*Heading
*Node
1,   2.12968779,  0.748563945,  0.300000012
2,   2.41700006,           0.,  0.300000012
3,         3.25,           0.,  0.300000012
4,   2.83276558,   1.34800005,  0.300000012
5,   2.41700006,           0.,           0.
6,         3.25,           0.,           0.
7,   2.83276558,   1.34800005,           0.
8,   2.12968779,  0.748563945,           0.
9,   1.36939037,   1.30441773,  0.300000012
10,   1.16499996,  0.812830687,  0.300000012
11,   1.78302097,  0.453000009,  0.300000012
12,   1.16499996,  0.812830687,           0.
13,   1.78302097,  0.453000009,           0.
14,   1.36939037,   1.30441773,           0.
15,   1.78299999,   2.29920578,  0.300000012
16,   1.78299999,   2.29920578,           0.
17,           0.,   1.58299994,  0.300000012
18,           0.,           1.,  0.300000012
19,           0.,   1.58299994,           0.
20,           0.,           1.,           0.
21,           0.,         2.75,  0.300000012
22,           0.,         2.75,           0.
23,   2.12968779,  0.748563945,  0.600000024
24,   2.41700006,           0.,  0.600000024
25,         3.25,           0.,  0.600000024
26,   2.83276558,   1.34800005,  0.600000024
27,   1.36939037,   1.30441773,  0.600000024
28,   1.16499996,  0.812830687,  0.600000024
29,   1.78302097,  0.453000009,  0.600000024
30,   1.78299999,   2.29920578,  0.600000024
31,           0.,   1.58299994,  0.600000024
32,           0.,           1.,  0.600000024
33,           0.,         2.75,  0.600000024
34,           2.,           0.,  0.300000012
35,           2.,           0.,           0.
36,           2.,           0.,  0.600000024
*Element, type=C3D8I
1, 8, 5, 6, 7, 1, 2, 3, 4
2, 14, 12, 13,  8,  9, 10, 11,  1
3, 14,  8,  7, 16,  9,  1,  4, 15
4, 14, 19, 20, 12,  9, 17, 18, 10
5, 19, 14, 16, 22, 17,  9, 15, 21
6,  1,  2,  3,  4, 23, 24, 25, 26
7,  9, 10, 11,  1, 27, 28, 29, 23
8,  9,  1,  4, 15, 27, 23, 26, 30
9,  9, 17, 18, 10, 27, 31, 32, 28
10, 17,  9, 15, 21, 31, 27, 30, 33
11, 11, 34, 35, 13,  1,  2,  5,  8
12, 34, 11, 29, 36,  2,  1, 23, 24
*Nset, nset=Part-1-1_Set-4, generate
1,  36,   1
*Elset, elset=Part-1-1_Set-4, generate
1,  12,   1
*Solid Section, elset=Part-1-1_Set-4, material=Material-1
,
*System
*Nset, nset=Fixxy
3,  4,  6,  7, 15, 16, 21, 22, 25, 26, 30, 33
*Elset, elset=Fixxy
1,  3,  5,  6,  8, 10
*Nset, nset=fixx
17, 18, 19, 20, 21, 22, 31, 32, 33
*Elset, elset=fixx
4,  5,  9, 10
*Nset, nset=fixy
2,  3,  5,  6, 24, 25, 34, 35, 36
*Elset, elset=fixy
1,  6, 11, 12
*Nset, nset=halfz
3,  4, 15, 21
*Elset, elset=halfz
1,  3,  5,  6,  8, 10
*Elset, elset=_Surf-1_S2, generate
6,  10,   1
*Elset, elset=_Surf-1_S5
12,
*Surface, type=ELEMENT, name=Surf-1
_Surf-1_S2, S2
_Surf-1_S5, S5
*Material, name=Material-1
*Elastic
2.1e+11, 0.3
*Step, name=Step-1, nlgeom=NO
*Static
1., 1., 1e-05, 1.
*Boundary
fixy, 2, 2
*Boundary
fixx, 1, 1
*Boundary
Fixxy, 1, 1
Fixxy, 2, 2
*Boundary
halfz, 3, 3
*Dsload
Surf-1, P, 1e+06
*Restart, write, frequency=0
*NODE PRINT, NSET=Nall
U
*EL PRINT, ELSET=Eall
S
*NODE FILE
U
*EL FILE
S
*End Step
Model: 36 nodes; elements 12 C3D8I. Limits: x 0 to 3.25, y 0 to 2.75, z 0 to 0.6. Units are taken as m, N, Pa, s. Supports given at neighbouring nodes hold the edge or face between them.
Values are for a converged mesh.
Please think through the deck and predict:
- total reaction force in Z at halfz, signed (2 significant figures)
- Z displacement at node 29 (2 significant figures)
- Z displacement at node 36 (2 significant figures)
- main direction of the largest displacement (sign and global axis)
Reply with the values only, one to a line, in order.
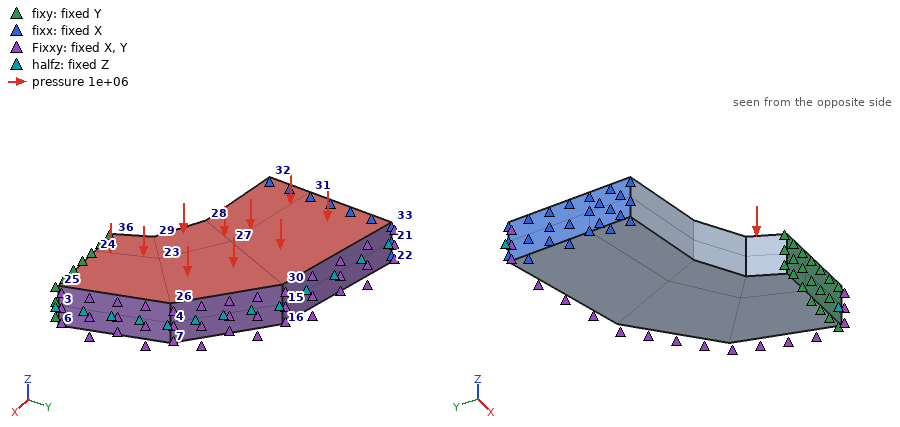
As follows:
5.2e+06 N
-1.0e-04 m
-8.6e-05 m
-Z
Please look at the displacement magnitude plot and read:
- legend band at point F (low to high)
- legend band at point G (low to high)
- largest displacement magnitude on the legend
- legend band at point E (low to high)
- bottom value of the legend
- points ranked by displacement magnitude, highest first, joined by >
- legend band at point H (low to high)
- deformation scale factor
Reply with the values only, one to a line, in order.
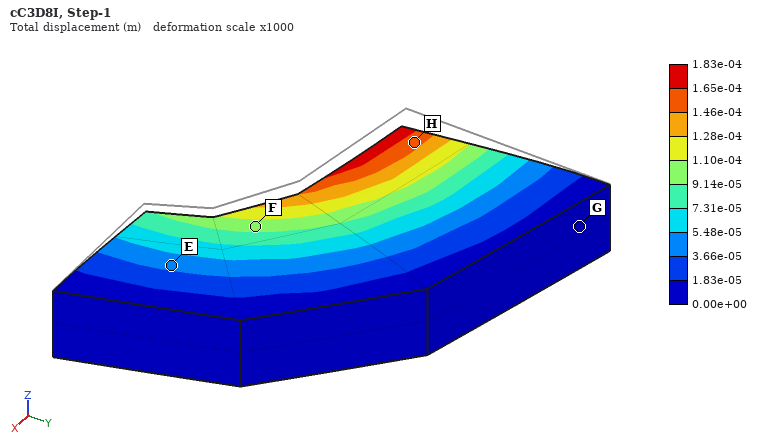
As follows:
9.14e-05 to 1.10e-04 m
0.00e+00 to 1.83e-05 m
1.83e-04 m
3.66e-05 to 5.48e-05 m
0.00e+00 m
H > F > E > G
1.46e-04 to 1.65e-04 m
1000
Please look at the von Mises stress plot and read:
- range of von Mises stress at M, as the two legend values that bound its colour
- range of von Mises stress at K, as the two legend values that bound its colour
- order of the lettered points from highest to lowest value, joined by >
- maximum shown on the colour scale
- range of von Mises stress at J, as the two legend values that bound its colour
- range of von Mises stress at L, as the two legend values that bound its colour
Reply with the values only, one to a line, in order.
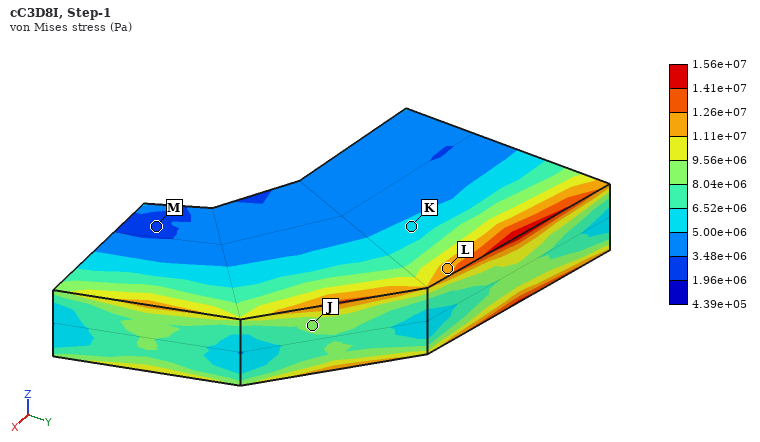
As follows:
1.96e+06 to 3.48e+06 Pa
5.00e+06 to 6.52e+06 Pa
L > J > K > M
1.56e+07 Pa
8.04e+06 to 9.56e+06 Pa
1.11e+07 to 1.26e+07 Pa
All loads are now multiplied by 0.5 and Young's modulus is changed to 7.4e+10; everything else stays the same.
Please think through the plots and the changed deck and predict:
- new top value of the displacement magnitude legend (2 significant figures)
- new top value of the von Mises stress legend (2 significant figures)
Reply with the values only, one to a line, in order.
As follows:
2.6e-04 m
7.8e+06 Pa
